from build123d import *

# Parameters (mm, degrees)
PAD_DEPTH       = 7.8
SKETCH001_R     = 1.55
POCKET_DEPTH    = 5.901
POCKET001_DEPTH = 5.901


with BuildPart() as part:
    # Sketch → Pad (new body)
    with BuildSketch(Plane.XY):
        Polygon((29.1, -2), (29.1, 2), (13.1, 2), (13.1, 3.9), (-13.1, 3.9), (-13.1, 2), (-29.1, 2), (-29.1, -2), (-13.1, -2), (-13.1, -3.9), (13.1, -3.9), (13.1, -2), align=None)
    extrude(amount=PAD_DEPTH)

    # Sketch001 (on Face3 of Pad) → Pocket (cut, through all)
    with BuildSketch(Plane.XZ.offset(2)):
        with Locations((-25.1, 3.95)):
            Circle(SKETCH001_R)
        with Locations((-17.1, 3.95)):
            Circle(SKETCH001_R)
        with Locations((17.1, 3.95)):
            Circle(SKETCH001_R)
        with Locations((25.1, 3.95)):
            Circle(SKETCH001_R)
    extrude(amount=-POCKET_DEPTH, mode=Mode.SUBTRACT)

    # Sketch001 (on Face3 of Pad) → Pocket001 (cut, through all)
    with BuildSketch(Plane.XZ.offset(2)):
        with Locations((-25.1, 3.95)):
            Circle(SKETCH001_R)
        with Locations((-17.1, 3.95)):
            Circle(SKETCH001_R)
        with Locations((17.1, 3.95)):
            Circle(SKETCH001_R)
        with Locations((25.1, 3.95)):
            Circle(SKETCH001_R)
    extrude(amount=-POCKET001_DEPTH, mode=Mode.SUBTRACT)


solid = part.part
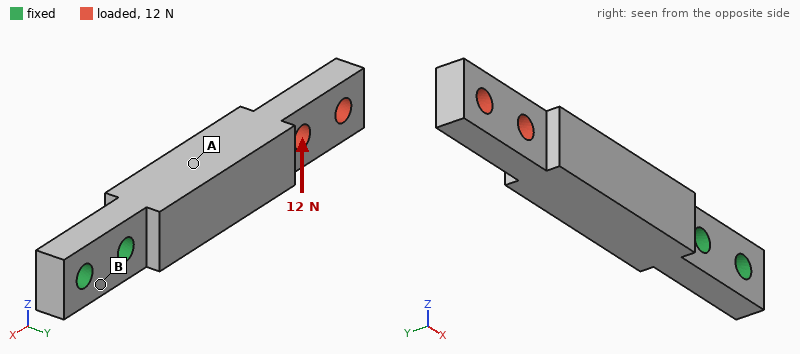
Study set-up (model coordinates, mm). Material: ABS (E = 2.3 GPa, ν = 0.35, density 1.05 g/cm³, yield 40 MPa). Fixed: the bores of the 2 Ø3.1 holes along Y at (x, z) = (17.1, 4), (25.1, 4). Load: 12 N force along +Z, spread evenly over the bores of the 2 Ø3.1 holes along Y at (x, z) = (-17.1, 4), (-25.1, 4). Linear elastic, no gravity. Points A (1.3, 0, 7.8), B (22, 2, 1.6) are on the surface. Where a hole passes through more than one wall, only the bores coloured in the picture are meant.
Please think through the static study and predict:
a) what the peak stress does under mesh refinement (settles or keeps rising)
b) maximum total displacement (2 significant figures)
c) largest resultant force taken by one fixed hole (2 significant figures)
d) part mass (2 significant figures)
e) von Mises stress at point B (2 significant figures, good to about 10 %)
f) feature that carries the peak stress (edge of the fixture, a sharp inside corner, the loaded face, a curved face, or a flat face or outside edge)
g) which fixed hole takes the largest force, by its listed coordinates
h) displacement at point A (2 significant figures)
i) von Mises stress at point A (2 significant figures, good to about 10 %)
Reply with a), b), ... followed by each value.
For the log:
a) keeps rising
b) 0.66 mm
c) 31 N
d) 2.6 g
e) 1.8 MPa
f) edge of the fixture
g) (17.1, 4)
h) 0.15 mm
i) 3.4 MPa
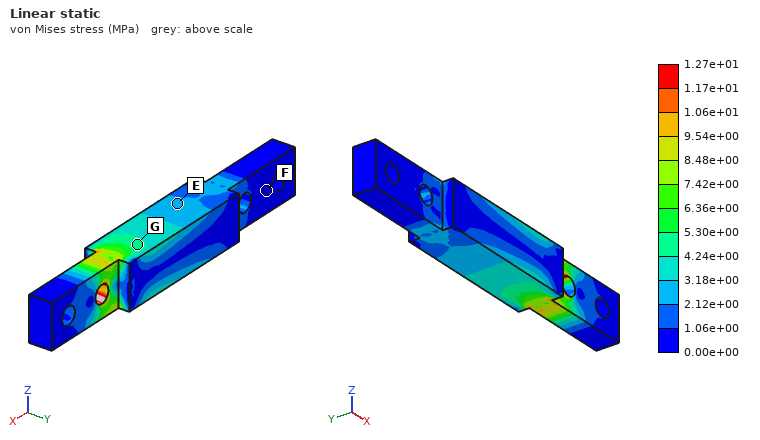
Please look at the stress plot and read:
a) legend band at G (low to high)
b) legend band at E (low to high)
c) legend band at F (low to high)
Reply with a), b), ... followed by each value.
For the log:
a) 4.24e+00 to 5.30e+00 MPa
b) 2.12e+00 to 3.18e+00 MPa
c) 0.00e+00 to 1.06e+00 MPa
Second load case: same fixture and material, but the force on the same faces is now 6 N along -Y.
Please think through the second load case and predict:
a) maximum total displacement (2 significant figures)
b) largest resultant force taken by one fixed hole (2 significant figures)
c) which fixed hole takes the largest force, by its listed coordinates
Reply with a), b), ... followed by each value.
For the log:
a) 0.60 mm
b) 9.2 N
c) (17.1, 4)
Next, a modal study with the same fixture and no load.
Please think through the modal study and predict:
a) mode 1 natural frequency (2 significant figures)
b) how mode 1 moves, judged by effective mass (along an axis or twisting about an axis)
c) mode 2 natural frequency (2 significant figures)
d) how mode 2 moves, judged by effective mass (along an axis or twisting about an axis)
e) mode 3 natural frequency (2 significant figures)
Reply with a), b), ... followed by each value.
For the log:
a) 660 Hz
b) along Y
c) 890 Hz
d) along Z
e) 3400 Hz
